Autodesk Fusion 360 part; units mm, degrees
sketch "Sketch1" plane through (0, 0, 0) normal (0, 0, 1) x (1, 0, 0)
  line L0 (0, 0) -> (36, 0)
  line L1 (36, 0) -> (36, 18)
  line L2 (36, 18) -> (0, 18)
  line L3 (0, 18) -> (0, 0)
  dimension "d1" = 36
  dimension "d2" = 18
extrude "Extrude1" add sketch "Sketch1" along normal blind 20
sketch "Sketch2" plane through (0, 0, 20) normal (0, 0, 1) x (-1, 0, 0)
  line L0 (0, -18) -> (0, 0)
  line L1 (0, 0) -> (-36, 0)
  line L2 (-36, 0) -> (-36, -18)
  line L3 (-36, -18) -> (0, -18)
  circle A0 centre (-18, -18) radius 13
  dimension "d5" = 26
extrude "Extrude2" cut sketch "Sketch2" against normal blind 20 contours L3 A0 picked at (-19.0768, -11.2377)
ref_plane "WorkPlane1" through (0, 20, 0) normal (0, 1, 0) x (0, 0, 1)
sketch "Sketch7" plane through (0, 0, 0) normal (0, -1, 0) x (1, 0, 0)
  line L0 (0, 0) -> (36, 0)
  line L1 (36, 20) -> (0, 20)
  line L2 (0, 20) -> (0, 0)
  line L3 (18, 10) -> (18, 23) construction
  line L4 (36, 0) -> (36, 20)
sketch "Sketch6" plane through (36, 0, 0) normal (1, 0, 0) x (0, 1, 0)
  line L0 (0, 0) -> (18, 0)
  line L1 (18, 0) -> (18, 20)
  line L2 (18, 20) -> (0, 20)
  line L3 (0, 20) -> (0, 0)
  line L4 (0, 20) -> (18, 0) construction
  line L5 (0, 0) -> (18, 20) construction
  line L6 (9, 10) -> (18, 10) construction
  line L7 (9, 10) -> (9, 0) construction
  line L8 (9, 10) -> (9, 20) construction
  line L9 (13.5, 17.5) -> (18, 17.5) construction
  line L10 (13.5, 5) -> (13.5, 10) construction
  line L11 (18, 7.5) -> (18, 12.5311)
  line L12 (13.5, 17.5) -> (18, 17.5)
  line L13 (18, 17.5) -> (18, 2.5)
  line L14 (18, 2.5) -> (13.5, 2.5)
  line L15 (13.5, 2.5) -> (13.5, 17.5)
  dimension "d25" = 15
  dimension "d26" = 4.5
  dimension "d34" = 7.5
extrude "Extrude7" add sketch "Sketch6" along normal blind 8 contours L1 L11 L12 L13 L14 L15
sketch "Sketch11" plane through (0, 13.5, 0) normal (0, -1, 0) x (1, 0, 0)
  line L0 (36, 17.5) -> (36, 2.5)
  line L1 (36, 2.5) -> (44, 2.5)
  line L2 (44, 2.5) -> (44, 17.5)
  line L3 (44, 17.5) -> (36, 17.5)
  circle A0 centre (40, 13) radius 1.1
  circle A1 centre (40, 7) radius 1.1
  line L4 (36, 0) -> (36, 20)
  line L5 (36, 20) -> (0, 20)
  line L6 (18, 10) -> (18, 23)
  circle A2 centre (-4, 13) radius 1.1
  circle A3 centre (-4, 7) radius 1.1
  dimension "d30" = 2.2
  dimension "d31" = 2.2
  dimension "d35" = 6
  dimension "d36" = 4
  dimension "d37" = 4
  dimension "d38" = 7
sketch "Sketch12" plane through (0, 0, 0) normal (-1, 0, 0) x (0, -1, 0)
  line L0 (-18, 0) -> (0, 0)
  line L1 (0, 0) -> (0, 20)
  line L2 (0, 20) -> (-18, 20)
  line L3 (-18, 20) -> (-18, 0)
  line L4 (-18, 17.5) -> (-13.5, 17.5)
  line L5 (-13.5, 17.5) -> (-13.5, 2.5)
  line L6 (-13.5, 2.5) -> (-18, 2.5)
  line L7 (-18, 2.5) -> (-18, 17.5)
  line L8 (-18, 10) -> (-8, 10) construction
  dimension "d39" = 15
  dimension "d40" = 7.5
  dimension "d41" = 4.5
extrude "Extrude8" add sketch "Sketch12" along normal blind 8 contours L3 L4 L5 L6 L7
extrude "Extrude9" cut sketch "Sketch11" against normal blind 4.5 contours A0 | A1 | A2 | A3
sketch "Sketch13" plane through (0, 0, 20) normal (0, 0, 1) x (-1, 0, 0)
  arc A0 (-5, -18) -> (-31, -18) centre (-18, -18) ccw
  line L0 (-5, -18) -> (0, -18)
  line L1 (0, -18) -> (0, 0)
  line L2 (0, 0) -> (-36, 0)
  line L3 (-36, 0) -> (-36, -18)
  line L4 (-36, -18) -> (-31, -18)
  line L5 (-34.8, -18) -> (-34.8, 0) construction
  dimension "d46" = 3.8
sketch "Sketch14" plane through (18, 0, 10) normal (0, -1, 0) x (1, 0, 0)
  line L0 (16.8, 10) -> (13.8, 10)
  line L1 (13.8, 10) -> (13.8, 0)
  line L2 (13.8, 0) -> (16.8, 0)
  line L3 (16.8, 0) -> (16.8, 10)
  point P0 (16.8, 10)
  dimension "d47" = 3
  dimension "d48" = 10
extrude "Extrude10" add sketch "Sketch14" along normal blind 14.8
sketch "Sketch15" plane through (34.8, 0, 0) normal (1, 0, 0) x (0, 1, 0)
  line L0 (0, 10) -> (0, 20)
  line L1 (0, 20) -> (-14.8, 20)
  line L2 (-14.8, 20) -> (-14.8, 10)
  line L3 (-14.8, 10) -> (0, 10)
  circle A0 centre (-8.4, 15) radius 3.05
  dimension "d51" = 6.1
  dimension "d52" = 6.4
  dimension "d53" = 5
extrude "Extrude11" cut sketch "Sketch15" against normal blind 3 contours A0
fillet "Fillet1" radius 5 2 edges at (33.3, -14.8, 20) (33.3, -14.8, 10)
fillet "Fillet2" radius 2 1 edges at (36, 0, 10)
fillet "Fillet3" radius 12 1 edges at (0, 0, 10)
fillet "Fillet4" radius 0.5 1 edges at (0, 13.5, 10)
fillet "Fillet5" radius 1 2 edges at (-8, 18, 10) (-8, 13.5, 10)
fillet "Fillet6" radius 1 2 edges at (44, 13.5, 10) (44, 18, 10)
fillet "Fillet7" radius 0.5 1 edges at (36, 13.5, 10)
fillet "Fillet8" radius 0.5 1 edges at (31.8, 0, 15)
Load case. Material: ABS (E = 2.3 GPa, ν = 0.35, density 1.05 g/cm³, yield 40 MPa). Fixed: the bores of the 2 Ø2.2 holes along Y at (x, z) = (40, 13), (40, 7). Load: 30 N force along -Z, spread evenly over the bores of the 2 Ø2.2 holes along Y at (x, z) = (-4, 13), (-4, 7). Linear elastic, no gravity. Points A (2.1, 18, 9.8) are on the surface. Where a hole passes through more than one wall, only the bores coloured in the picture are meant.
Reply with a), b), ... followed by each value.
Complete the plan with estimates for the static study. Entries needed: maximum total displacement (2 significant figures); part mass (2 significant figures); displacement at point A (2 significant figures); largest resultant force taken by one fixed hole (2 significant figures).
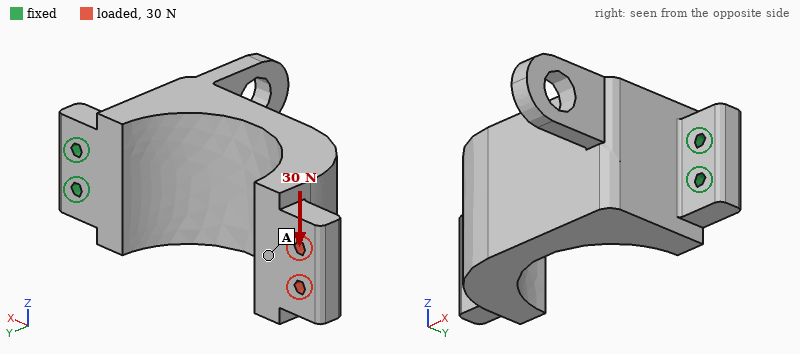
a) 0.65 mm
b) 8.8 g
c) 0.51 mm
d) 170 N
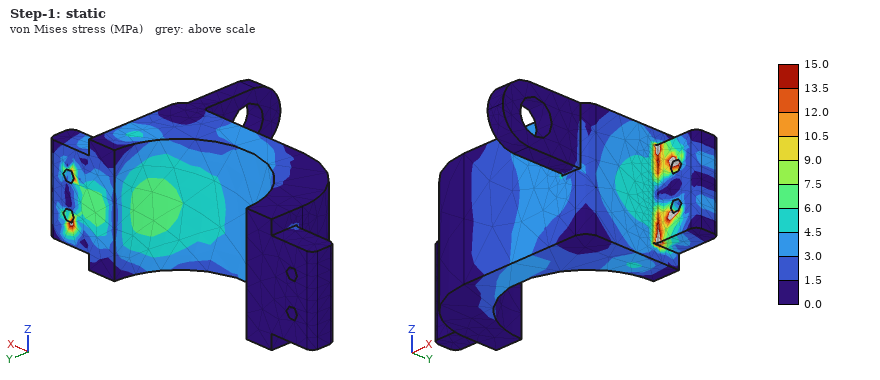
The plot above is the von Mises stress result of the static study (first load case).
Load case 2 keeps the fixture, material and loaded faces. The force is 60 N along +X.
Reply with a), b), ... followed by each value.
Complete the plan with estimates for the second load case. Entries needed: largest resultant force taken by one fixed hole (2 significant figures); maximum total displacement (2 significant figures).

a) 30 N
b) 0.77 mm
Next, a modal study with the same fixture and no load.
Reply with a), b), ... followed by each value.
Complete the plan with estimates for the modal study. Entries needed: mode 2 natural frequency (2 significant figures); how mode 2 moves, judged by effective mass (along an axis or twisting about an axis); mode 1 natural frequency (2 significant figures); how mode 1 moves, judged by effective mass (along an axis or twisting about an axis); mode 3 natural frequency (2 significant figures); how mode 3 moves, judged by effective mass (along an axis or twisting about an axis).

a) 800 Hz
b) along Z
c) 410 Hz
d) along Y
e) 1400 Hz
f) along X
